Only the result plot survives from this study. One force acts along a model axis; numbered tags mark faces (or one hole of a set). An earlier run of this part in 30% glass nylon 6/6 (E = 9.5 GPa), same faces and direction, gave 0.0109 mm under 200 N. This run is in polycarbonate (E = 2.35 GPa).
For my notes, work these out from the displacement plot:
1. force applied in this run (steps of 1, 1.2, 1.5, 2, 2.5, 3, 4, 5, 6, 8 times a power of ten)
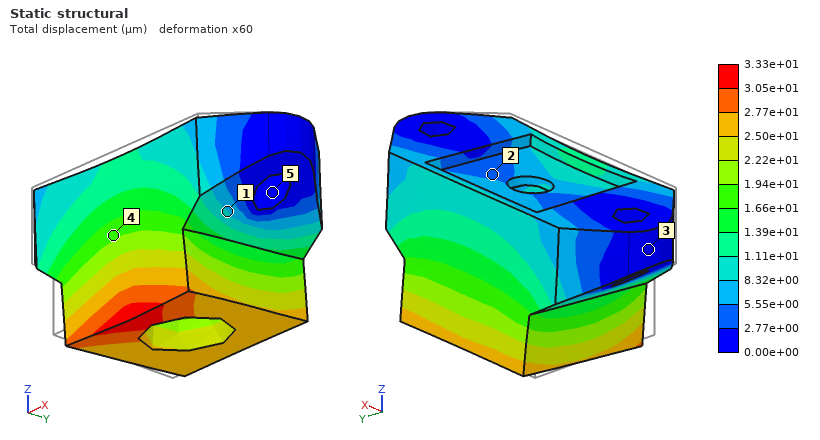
150 N
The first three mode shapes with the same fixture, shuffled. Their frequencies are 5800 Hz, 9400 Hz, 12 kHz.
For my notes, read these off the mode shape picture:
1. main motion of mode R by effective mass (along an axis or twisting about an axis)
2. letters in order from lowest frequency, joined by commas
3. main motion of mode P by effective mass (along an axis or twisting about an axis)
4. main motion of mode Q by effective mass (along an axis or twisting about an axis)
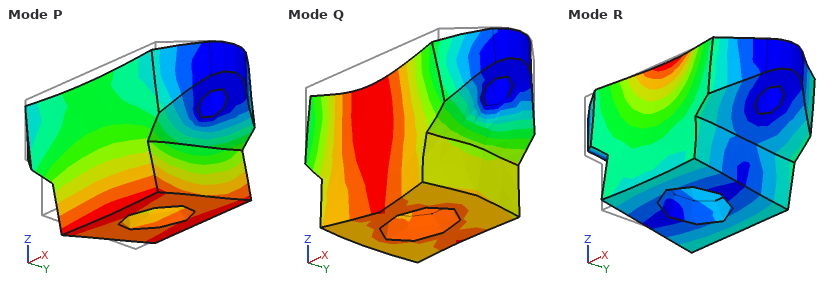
along Y
P, Q, R
along Y
along Z
